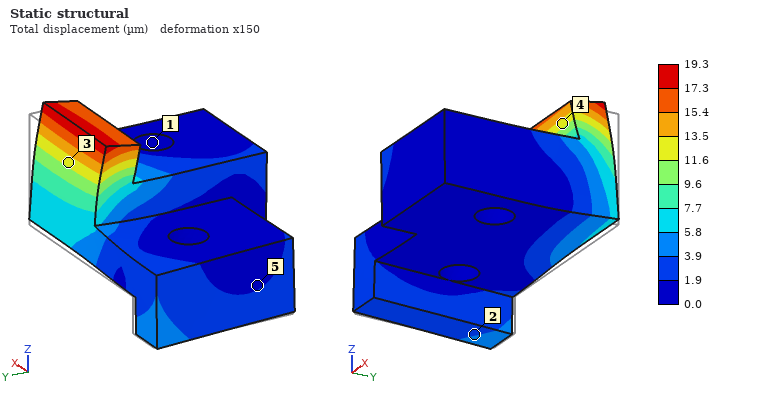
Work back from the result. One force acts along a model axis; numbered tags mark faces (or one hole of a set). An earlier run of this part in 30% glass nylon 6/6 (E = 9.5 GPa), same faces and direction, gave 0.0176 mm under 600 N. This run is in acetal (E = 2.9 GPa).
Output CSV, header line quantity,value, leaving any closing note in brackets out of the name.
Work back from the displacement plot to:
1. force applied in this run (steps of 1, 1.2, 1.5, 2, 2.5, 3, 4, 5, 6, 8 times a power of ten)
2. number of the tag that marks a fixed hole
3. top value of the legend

quantity,value
force applied in this run,200 N
number of the tag that marks a fixed hole,1
top value of the legend,19.3 µm
